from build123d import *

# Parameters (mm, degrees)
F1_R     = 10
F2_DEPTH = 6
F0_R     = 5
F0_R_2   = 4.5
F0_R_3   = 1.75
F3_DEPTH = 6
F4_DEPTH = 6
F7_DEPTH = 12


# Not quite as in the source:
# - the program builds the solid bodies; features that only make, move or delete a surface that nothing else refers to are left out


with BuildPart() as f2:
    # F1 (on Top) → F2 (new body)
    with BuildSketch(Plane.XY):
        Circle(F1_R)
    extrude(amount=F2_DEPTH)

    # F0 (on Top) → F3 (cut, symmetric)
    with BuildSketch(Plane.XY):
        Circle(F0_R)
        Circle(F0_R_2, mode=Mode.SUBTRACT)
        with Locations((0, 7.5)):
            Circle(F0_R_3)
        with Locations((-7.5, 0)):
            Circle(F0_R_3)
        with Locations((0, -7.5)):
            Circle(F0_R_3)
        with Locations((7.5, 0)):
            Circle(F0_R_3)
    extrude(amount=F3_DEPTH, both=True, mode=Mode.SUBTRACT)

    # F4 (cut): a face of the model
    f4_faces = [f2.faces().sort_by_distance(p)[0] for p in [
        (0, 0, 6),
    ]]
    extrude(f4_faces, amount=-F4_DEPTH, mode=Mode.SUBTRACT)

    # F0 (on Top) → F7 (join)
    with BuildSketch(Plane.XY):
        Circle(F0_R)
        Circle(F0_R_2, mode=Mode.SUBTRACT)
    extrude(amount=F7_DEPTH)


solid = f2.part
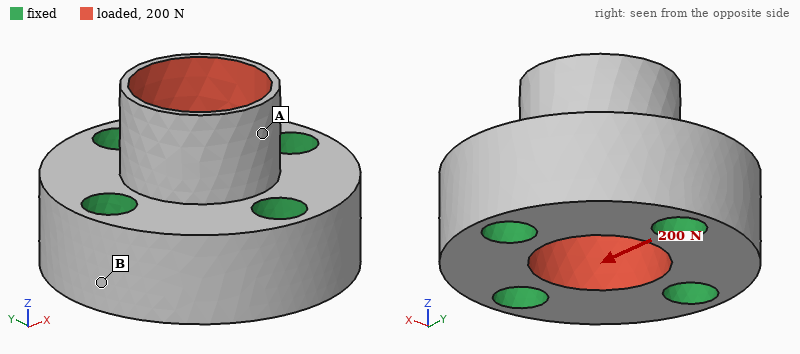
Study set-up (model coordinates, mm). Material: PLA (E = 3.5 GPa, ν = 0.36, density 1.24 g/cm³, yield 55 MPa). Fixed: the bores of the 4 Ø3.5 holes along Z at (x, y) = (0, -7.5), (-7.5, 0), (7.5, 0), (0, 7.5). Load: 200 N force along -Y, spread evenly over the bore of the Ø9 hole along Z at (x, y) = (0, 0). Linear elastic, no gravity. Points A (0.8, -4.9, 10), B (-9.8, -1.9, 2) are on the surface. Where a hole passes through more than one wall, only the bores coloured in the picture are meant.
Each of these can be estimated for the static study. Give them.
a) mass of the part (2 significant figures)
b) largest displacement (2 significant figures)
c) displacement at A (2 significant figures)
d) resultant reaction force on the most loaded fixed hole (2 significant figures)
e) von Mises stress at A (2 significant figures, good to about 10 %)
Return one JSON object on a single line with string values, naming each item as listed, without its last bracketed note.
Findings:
{"mass of the part": "1.7 g", "largest displacement": "50 µm", "displacement at A": "43 µm", "resultant reaction force on the most loaded fixed hole": "60 N", "von Mises stress at A": "6.0 MPa"}
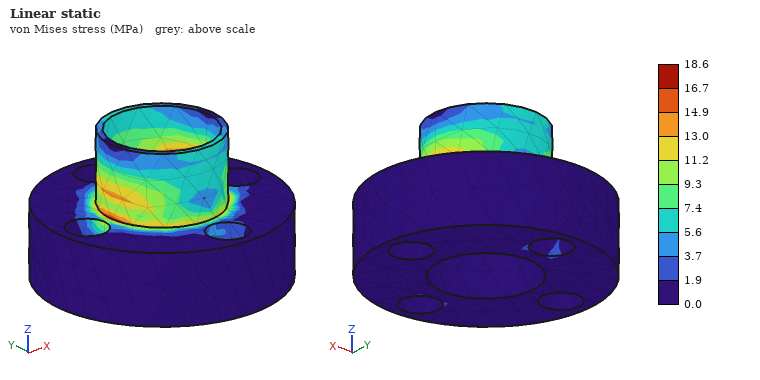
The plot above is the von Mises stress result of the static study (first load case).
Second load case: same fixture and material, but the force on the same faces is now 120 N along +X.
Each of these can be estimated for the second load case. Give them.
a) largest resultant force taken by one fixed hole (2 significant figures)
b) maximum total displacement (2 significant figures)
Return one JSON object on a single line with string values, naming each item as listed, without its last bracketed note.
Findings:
{"largest resultant force taken by one fixed hole": "36 N", "maximum total displacement": "30 µm"}
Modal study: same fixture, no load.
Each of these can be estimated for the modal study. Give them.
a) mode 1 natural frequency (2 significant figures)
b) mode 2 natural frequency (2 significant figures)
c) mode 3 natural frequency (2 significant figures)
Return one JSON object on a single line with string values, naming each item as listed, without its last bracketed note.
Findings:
{"mode 1 natural frequency": "16 kHz", "mode 2 natural frequency": "16 kHz", "mode 3 natural frequency": "19 kHz"}
